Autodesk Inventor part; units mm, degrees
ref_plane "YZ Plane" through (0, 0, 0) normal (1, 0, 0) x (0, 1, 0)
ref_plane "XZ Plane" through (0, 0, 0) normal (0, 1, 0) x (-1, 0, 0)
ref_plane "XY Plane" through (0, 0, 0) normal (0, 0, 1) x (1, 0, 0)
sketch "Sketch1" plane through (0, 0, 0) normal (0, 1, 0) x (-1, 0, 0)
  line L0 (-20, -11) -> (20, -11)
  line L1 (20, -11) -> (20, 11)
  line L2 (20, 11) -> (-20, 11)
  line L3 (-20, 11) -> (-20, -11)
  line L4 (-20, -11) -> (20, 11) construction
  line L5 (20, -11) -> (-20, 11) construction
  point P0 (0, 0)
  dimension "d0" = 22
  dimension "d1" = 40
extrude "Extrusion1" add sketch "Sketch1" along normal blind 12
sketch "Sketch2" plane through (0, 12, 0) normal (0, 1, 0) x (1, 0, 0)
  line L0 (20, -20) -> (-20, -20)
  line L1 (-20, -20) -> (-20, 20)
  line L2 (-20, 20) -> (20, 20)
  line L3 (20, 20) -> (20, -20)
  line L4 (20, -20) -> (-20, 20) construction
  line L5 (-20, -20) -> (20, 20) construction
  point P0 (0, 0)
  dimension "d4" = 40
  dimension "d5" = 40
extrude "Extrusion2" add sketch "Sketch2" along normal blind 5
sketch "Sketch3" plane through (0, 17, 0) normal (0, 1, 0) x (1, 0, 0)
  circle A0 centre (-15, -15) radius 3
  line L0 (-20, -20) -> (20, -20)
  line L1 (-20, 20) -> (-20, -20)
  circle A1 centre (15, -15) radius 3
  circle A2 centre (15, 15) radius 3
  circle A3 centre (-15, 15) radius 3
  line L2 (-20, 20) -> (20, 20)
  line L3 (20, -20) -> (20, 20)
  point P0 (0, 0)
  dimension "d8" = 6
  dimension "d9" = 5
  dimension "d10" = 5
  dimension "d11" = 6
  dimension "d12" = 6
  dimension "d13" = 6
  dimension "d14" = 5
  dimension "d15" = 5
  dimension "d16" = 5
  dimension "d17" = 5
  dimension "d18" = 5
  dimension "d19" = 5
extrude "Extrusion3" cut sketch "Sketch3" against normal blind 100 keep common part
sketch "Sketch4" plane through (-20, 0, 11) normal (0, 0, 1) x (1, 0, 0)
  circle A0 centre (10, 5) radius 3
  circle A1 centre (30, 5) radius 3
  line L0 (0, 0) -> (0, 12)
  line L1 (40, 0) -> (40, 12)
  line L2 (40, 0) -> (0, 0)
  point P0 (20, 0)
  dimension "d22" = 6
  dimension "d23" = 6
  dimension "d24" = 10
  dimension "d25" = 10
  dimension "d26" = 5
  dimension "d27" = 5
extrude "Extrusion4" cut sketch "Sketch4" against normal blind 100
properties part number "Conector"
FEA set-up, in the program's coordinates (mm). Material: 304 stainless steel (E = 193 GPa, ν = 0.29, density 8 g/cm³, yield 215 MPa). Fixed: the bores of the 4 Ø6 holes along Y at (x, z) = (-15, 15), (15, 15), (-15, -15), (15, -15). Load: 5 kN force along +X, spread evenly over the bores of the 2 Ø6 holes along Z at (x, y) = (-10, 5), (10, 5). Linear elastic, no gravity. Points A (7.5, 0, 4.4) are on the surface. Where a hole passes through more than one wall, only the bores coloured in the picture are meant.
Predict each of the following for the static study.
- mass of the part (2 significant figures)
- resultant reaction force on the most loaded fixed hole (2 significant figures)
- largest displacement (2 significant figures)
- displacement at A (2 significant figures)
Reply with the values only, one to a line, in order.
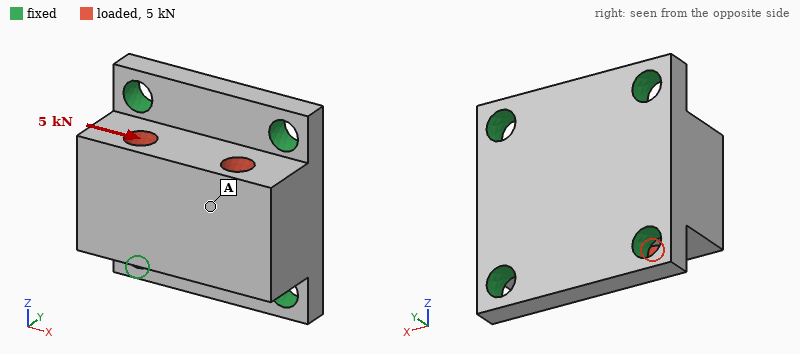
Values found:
130 g
1.6 kN
4.2 µm
3.4 µm
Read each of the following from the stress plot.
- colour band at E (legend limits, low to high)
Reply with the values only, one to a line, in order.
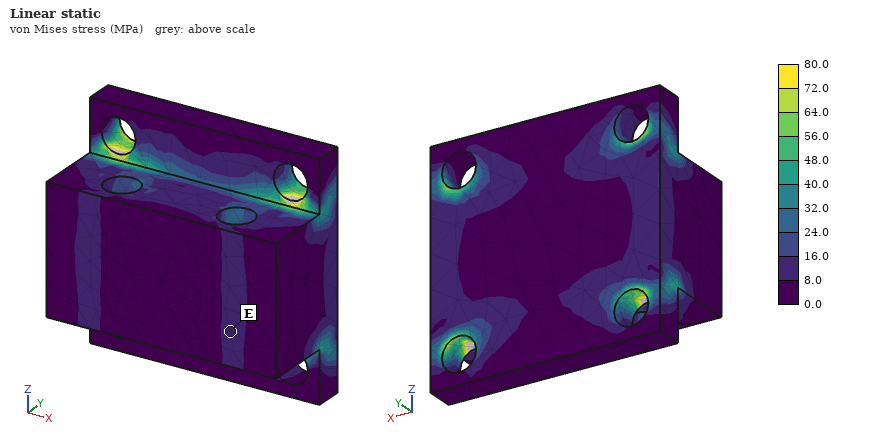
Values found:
8.0 to 16.0 MPa
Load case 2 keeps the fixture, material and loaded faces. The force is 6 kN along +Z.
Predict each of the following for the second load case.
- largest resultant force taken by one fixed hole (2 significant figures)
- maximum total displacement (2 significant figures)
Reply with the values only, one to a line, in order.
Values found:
1.9 kN
4.1 µm
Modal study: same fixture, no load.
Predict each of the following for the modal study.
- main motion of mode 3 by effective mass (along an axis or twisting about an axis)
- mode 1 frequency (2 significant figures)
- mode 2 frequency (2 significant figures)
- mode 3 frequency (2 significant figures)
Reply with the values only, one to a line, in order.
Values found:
along Z
22 kHz
22 kHz
26 kHz
